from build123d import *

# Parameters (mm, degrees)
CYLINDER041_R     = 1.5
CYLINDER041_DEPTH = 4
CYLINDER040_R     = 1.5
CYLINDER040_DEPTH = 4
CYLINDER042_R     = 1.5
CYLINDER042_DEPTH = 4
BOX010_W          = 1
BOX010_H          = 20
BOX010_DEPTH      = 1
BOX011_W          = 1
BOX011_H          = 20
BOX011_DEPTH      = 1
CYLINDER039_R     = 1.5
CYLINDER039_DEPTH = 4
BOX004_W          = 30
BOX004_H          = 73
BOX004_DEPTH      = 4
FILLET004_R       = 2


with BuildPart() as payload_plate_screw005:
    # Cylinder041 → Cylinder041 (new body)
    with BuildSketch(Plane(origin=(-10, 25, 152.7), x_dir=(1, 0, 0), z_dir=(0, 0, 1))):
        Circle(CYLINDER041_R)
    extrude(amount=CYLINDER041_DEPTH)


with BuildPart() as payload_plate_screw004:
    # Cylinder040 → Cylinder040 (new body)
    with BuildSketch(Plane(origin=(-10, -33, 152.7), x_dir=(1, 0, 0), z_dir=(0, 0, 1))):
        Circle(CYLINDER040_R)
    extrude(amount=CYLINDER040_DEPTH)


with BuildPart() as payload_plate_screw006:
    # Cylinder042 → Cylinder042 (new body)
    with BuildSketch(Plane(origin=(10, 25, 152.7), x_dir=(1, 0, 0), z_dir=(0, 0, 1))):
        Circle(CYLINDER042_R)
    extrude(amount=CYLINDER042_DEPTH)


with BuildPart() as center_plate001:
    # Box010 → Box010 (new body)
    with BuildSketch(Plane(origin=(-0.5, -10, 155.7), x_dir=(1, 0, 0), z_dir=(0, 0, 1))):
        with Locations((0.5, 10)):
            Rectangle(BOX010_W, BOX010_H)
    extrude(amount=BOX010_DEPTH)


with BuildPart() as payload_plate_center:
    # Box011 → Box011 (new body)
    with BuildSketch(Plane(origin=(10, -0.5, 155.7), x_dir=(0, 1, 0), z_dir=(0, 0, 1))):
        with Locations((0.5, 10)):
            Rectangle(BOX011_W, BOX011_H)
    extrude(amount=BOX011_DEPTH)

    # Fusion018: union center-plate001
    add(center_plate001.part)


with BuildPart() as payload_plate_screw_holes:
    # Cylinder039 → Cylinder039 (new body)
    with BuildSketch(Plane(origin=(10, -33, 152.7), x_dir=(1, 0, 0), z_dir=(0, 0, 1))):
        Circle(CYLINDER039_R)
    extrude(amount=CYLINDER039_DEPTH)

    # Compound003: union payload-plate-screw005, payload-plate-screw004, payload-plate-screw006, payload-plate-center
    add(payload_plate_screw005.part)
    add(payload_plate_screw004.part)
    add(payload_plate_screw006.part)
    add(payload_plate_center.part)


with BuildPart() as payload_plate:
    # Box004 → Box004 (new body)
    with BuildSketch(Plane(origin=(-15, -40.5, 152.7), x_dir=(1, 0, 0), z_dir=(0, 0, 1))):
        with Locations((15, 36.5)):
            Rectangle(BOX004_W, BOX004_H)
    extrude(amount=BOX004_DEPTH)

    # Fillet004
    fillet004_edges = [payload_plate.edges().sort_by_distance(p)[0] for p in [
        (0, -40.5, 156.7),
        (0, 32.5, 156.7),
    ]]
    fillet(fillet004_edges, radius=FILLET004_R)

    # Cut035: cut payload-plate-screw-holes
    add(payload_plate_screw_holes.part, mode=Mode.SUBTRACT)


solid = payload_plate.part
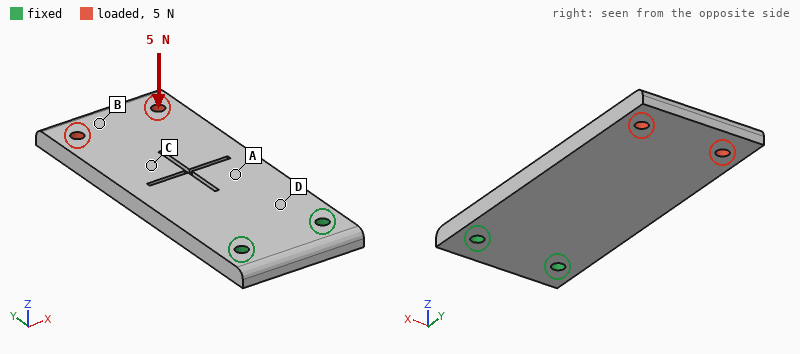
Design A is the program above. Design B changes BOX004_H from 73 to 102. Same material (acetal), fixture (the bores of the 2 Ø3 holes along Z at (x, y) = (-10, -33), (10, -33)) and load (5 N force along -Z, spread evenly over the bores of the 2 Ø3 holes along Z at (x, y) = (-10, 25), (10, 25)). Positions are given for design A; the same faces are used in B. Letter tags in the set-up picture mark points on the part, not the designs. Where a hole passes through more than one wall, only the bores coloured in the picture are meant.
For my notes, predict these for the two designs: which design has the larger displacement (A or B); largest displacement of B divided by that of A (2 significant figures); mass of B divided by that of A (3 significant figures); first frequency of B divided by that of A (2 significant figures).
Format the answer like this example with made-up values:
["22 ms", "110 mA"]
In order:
["B", "1.3", "1.41", "0.67"]
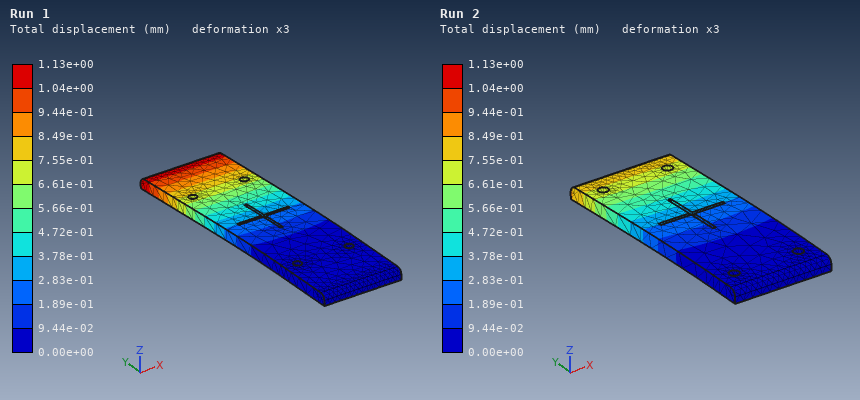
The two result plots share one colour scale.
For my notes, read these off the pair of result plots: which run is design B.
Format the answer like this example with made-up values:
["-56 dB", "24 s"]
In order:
["Run 1"]
